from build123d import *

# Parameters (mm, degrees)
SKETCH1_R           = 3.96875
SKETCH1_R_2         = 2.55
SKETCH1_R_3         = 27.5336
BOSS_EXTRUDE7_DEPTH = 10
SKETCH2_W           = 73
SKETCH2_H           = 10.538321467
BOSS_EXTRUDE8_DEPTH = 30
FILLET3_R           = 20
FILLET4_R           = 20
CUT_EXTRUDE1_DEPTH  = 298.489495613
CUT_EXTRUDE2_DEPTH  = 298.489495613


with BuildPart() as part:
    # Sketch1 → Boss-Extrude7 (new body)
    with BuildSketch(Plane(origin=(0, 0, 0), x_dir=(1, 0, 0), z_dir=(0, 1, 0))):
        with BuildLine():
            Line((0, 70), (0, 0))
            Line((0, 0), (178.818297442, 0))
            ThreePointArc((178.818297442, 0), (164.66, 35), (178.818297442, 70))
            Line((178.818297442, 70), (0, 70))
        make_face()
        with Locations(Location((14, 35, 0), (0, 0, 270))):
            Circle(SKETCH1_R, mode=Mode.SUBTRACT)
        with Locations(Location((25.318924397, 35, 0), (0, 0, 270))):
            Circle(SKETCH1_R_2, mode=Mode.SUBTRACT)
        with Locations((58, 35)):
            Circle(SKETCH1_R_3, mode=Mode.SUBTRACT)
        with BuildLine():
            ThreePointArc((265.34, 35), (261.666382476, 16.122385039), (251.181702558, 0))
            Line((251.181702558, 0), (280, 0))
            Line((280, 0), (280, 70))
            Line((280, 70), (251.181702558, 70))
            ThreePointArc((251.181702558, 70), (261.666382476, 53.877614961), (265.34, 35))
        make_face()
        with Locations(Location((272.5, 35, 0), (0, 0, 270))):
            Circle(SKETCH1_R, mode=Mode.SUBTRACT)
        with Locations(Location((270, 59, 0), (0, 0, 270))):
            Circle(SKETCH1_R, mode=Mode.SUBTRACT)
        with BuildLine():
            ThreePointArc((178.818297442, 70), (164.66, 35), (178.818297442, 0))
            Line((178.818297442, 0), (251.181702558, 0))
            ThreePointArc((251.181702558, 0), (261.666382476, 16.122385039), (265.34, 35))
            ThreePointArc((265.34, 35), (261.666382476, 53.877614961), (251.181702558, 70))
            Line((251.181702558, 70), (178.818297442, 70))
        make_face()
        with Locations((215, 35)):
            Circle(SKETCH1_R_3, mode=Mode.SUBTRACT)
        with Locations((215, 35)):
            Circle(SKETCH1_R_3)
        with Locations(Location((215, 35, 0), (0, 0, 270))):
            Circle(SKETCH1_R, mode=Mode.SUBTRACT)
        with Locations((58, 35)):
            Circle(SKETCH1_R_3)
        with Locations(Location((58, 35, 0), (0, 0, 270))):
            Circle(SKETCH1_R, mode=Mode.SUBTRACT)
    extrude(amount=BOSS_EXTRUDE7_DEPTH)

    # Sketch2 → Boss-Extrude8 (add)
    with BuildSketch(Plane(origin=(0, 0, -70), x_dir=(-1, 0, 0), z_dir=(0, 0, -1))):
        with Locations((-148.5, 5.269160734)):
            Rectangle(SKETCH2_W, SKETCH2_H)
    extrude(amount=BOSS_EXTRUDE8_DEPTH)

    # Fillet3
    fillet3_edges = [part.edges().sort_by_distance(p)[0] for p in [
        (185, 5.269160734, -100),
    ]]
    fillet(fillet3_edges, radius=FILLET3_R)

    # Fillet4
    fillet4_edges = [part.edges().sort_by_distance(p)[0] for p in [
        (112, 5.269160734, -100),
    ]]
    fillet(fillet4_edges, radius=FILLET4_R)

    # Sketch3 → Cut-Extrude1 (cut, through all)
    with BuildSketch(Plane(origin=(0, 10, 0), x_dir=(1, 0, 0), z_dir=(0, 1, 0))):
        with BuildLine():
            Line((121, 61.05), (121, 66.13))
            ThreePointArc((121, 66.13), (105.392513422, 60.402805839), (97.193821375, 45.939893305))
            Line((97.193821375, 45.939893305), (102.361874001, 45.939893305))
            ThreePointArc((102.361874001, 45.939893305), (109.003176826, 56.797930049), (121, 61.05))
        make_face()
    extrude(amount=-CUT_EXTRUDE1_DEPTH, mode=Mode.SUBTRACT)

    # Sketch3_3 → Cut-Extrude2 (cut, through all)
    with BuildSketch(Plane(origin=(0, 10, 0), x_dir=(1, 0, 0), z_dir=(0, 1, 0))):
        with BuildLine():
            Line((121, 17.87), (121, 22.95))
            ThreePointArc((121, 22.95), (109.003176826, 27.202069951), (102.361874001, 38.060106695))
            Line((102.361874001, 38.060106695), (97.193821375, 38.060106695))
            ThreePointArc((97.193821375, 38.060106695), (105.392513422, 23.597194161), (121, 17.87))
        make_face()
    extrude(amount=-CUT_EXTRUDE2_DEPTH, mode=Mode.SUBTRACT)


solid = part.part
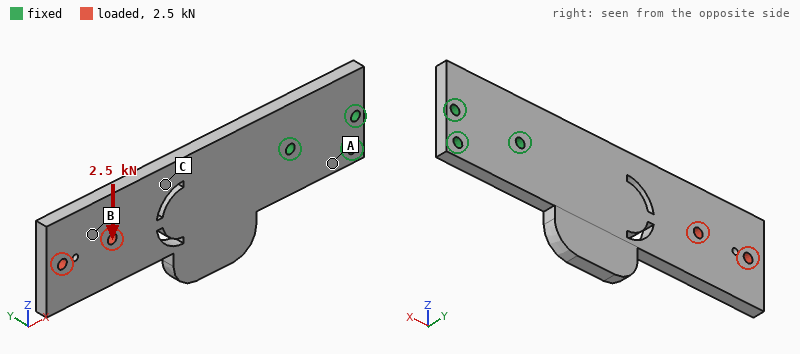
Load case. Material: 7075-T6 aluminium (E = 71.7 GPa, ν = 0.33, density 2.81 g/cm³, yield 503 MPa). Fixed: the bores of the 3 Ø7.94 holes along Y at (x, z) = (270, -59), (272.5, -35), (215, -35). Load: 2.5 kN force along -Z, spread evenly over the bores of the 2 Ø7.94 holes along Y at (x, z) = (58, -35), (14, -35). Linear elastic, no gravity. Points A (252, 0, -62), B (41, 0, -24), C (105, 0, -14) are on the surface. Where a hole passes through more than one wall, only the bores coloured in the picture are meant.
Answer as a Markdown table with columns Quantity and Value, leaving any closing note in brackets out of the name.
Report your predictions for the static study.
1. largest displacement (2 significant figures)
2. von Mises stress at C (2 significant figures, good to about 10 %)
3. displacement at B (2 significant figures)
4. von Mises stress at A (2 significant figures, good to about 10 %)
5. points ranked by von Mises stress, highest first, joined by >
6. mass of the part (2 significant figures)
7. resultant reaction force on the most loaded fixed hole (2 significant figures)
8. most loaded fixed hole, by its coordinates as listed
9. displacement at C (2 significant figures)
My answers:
| Quantity | Value |
|---|---|
| largest displacement | 0.50 mm |
| von Mises stress at C | 13 MPa |
| displacement at B | 0.38 mm |
| von Mises stress at A | 25 MPa |
| points ranked by von Mises stress, highest first, joined by > | A > C > B |
| mass of the part | 590 g |
| resultant reaction force on the most loaded fixed hole | 8.4 kN |
| most loaded fixed hole, by its coordinates as listed | (215, -35) |
| displacement at C | 0.22 mm |
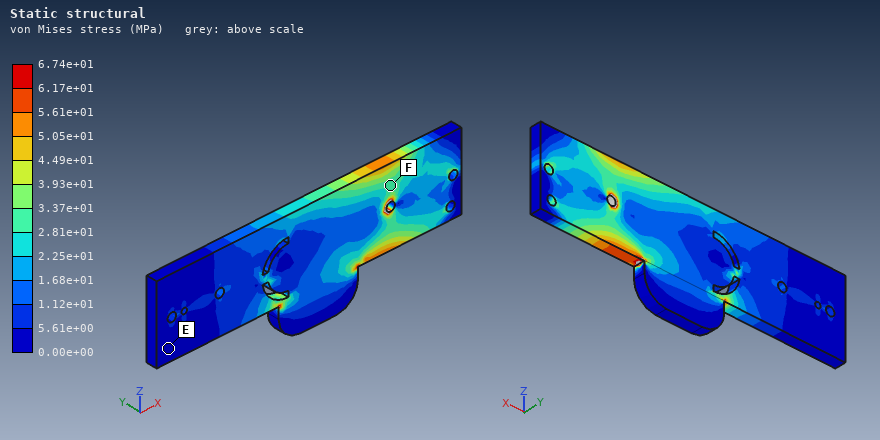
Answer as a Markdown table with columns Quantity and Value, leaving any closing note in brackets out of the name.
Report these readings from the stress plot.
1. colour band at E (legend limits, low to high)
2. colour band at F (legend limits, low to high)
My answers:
| Quantity | Value |
|---|---|
| colour band at E | 0.00e+00 to 5.61e+00 MPa |
| colour band at F | 2.81e+01 to 3.37e+01 MPa |
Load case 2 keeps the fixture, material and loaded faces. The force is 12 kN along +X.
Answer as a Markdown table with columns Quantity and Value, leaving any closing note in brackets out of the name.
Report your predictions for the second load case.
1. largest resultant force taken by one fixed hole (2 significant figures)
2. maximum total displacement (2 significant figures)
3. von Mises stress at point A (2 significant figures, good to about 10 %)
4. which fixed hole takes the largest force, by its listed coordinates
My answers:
| Quantity | Value |
|---|---|
| largest resultant force taken by one fixed hole | 8.8 kN |
| maximum total displacement | 62 µm |
| von Mises stress at point A | 7.5 MPa |
| which fixed hole takes the largest force, by its listed coordinates | (215, -35) |
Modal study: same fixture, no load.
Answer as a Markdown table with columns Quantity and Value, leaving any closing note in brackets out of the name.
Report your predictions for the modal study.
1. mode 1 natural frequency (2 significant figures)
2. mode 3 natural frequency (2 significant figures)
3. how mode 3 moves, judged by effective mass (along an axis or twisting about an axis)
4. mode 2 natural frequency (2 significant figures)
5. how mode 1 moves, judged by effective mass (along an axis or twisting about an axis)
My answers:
| Quantity | Value |
|---|---|
| mode 1 natural frequency | 180 Hz |
| mode 3 natural frequency | 900 Hz |
| how mode 3 moves, judged by effective mass | along Z |
| mode 2 natural frequency | 780 Hz |
| how mode 1 moves, judged by effective mass | along Y |
